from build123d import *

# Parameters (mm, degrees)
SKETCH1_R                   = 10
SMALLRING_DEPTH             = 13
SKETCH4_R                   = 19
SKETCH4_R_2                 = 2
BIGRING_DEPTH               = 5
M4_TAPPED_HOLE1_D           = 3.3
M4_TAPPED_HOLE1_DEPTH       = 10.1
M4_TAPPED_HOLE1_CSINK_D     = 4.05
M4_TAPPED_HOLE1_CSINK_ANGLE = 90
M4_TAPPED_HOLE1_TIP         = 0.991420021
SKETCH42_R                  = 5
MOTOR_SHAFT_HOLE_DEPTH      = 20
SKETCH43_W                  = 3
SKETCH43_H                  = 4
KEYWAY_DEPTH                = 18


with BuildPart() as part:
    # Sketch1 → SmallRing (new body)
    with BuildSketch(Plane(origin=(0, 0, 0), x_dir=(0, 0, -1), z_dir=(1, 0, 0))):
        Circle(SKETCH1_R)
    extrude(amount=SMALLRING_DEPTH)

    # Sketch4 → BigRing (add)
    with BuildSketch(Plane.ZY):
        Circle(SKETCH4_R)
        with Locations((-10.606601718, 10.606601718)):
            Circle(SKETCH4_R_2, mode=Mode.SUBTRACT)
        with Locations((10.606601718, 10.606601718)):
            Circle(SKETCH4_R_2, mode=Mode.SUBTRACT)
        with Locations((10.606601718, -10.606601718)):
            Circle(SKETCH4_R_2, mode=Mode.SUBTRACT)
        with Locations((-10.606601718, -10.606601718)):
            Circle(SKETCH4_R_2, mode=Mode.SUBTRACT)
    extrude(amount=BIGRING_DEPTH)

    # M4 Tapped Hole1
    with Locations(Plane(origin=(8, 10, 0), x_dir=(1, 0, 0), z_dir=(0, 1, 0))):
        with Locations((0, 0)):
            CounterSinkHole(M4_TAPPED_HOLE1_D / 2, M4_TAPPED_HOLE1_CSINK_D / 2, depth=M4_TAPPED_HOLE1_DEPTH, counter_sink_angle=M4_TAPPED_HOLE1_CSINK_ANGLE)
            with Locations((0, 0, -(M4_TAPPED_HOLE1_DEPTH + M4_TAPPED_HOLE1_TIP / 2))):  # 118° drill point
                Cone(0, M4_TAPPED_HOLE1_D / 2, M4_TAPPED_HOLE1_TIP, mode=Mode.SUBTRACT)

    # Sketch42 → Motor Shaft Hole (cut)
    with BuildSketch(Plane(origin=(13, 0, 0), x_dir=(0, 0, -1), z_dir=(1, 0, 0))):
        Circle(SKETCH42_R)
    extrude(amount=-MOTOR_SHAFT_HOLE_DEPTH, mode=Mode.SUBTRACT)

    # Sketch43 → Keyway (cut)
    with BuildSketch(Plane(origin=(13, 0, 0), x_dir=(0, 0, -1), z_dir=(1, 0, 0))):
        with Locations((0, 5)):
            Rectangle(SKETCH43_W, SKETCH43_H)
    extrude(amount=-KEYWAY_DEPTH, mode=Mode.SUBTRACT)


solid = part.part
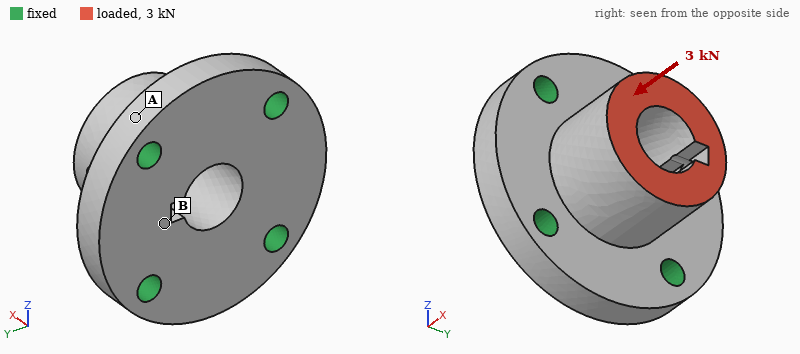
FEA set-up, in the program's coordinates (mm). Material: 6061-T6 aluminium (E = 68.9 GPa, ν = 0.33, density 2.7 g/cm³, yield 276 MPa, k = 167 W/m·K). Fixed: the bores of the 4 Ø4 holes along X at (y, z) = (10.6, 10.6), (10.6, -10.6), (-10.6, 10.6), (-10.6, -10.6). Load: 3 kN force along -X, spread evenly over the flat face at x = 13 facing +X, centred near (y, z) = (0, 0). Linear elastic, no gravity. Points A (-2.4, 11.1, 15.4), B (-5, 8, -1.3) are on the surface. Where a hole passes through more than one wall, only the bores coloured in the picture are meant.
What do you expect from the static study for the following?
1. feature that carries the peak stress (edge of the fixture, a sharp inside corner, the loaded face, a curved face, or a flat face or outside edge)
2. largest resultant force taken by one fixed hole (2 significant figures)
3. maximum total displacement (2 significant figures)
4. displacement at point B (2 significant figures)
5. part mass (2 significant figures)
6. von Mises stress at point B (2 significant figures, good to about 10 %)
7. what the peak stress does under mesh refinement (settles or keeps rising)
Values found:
edge of the fixture
800 N
8.6 µm
5.5 µm
21 g
18 MPa
keeps rising
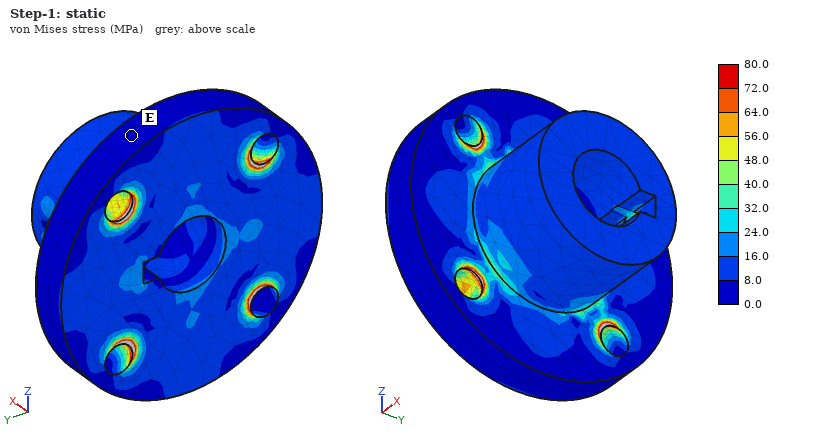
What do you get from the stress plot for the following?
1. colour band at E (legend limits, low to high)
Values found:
0.0 to 8.0 MPa
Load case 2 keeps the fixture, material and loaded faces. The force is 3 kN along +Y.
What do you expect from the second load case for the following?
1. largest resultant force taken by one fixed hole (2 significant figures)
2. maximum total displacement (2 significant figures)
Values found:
1.4 kN
38 µm
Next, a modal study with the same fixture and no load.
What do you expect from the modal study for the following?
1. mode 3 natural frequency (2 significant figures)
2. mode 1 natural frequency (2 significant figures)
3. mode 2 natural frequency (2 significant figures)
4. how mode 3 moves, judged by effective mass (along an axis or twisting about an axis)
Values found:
32 kHz
25 kHz
25 kHz
along X
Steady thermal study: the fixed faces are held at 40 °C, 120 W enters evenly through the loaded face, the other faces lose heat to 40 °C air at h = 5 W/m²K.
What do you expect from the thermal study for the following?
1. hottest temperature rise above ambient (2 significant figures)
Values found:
63 K
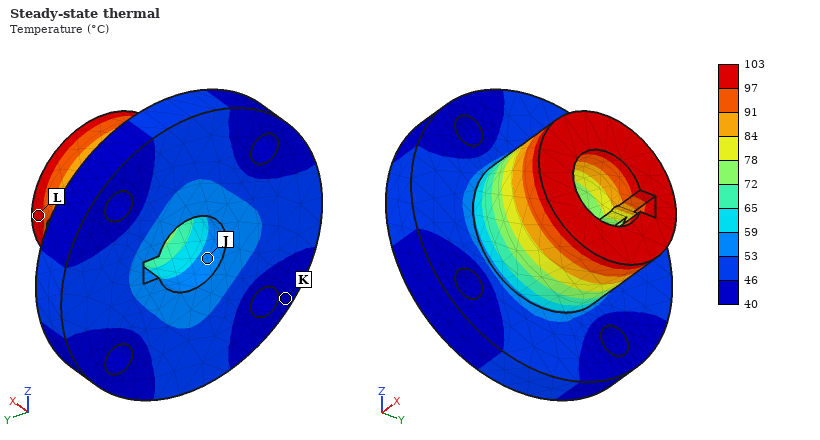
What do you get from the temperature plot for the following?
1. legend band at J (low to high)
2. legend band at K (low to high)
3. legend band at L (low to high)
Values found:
53 to 59 °C
40 to 46 °C
97 to 103 °C
